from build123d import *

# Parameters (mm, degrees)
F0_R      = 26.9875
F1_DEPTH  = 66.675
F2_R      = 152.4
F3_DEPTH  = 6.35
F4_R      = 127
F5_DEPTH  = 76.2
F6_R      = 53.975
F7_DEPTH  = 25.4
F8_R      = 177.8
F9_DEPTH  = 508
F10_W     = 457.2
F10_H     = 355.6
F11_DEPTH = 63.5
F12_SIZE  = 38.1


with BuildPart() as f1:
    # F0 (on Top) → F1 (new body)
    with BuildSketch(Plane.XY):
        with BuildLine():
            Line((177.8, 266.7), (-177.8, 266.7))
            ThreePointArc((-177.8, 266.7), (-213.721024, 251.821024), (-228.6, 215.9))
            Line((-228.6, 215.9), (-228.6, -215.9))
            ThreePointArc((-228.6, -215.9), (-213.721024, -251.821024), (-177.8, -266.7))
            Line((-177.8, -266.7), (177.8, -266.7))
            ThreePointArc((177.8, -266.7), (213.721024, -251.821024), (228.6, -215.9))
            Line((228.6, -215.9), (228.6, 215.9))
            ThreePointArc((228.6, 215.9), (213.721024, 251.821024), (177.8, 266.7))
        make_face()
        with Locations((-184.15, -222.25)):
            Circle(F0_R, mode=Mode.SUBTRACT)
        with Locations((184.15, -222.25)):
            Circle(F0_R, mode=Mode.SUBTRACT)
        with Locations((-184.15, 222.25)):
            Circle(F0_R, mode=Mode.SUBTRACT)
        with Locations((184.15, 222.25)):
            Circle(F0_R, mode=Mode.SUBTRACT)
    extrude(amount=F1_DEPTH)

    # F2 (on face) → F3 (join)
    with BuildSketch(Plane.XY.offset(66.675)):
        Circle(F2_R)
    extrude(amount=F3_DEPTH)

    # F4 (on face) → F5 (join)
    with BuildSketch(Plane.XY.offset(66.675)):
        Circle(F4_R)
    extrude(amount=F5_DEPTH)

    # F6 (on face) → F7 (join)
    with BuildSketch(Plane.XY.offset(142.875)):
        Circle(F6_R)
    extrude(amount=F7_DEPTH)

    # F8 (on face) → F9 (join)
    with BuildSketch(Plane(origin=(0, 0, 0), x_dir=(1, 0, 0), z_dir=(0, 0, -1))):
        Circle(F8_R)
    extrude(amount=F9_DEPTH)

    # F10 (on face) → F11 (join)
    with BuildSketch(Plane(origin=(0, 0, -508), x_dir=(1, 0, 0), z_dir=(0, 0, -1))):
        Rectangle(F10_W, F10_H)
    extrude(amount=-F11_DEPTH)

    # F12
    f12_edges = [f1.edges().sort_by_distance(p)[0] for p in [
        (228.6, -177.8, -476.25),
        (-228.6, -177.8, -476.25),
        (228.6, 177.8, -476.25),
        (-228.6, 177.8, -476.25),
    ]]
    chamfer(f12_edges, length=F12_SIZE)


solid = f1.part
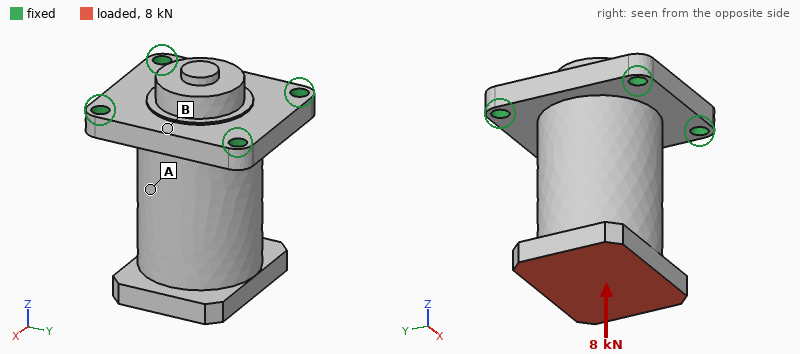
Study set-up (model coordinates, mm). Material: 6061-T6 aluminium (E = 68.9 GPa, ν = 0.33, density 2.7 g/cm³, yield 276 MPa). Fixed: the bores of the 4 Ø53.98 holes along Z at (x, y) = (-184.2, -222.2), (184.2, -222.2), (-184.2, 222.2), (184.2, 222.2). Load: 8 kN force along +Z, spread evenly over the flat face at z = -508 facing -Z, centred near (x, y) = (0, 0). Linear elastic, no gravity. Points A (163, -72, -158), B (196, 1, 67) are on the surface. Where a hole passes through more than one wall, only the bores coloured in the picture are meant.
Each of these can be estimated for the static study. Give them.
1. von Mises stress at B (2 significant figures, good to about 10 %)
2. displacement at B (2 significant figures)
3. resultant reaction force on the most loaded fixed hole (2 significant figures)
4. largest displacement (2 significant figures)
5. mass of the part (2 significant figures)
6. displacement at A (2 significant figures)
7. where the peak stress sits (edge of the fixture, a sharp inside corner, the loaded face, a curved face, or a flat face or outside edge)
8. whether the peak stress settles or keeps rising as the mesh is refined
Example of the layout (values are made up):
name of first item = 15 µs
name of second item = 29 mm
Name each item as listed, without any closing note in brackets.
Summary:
von Mises stress at B = 0.27 MPa
displacement at B = 2.2 µm
resultant reaction force on the most loaded fixed hole = 2.0 kN
largest displacement = 3.5 µm
mass of the part = 200 kg
displacement at A = 2.3 µm
where the peak stress sits = edge of the fixture
whether the peak stress settles or keeps rising as the mesh is refined = keeps rising
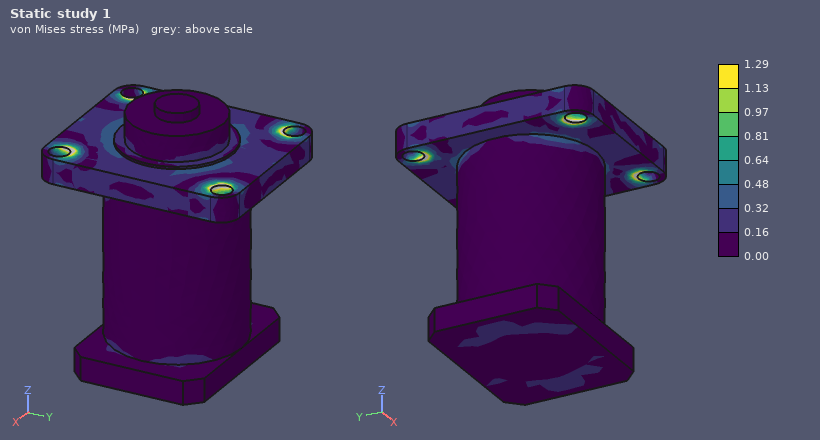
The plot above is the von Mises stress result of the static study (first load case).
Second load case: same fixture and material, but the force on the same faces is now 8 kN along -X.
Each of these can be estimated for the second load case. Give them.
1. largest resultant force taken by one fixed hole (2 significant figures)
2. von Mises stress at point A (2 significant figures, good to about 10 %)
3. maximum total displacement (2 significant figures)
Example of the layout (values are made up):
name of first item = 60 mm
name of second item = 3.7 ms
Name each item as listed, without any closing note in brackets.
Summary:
largest resultant force taken by one fixed hole = 7.0 kN
von Mises stress at point A = 0.56 MPa
maximum total displacement = 40 µm
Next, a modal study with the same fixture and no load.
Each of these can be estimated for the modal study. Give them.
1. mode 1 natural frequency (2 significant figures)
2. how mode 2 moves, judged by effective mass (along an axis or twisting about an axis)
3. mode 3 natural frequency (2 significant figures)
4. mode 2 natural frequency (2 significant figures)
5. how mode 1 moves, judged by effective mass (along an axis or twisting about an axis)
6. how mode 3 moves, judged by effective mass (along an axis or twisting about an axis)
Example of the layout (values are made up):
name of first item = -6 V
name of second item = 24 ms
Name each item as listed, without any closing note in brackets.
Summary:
mode 1 natural frequency = 310 Hz
how mode 2 moves, judged by effective mass = along Y
mode 3 natural frequency = 690 Hz
mode 2 natural frequency = 360 Hz
how mode 1 moves, judged by effective mass = along X
how mode 3 moves, judged by effective mass = along Z
